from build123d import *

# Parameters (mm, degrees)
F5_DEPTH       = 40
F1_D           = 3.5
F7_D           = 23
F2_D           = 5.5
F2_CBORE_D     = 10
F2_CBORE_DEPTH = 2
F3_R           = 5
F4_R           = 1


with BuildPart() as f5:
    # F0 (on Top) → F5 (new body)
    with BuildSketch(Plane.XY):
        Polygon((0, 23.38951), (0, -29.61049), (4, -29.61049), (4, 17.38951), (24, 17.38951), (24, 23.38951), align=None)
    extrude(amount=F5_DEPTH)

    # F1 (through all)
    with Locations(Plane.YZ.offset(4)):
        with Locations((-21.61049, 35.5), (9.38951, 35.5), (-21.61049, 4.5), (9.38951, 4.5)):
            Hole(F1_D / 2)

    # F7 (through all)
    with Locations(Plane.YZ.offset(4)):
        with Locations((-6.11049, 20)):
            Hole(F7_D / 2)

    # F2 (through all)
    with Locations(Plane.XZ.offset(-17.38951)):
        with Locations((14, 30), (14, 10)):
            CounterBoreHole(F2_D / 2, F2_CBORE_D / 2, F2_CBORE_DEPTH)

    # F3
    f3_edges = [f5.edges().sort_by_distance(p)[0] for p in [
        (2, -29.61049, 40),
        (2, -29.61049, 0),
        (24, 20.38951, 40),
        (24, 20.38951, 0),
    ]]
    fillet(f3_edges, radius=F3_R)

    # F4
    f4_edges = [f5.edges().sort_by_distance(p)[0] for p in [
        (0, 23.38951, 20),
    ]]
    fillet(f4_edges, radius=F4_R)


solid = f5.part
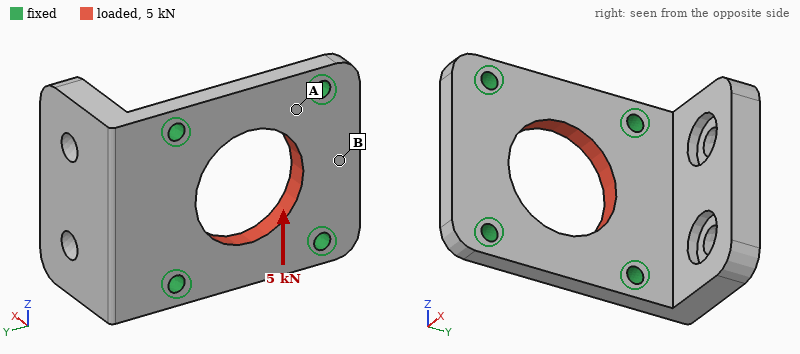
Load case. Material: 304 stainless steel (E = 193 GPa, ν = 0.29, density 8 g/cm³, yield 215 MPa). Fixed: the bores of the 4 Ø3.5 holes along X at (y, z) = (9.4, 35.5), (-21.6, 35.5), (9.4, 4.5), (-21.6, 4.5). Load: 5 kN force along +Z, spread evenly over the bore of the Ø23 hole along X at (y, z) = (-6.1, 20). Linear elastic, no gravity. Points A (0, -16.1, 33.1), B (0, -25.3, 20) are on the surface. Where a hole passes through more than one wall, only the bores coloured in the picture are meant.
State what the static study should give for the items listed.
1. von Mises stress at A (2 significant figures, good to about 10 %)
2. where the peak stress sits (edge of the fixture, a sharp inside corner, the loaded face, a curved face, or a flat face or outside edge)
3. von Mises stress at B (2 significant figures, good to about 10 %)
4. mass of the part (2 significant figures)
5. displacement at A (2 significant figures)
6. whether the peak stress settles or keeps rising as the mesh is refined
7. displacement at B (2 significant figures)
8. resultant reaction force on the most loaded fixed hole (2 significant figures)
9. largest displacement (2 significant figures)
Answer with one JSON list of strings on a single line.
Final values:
["28 MPa", "edge of the fixture", "13 MPa", "87 g", "1.7 µm", "keeps rising", "0.86 µm", "1.3 kN", "4.4 µm"]
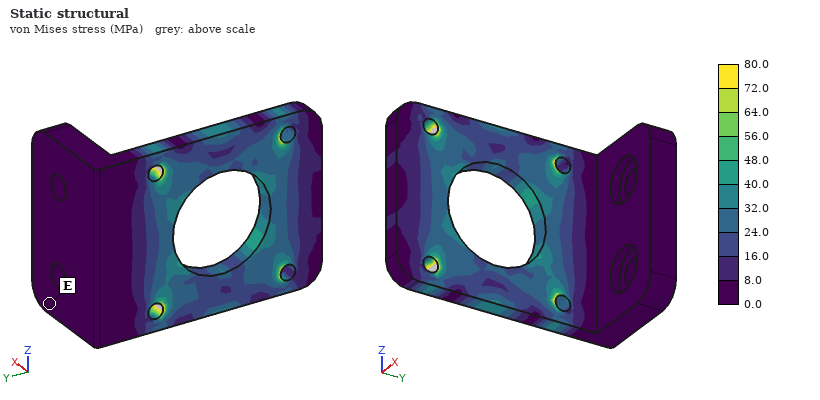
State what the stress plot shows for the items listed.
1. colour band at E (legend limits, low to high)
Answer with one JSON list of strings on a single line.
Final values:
["0.0 to 8.0 MPa"]
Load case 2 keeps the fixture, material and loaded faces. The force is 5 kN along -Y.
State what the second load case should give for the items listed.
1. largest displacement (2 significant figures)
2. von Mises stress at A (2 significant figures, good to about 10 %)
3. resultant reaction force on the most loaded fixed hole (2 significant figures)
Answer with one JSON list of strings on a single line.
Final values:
["3.7 µm", "25 MPa", "1.3 kN"]
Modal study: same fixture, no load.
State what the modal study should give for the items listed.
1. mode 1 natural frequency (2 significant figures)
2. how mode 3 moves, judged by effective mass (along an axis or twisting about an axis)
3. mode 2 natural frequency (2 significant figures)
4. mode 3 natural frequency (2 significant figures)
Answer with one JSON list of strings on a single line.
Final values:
["3300 Hz", "along X", "7700 Hz", "12 kHz"]
